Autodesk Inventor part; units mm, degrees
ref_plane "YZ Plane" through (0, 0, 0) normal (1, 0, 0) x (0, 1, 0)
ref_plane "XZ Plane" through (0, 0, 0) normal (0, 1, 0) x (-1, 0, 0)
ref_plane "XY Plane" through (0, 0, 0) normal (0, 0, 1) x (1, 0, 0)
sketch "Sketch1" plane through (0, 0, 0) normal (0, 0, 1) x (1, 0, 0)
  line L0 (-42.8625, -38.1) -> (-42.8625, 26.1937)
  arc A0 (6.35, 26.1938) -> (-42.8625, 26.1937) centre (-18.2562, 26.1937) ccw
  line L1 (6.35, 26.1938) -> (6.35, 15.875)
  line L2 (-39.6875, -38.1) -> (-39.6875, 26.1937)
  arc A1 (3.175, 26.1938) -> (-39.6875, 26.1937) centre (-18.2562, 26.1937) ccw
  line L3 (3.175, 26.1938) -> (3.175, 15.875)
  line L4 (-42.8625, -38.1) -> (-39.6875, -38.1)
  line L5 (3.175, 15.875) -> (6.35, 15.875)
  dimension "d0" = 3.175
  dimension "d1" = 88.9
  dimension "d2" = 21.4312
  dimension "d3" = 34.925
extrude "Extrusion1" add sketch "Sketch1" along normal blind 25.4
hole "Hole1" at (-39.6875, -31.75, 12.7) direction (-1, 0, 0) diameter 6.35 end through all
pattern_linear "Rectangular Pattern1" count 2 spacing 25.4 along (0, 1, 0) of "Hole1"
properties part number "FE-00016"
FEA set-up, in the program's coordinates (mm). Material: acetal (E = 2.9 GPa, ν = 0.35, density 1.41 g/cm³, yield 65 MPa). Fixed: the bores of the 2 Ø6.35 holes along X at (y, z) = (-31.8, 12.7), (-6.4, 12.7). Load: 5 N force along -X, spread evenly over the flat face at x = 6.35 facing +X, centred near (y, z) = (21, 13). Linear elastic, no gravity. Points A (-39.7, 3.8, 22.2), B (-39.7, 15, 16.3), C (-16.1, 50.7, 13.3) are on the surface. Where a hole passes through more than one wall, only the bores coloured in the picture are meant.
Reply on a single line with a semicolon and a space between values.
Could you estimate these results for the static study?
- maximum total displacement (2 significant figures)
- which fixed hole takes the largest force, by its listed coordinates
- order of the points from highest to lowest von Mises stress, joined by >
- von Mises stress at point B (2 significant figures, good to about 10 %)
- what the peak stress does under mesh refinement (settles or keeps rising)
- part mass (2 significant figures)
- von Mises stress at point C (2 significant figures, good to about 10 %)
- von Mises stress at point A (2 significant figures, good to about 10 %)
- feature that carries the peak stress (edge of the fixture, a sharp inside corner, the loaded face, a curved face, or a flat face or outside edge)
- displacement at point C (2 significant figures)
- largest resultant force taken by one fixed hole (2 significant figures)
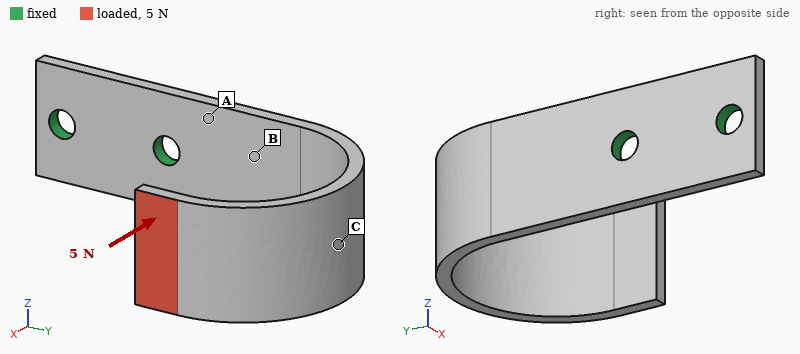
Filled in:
1.2 mm; (-6.4, 12.7); C > A > B; 0.63 MPa; keeps rising; 16 g; 2.7 MPa; 1.9 MPa; edge of the fixture; 0.26 mm; 5.6 N
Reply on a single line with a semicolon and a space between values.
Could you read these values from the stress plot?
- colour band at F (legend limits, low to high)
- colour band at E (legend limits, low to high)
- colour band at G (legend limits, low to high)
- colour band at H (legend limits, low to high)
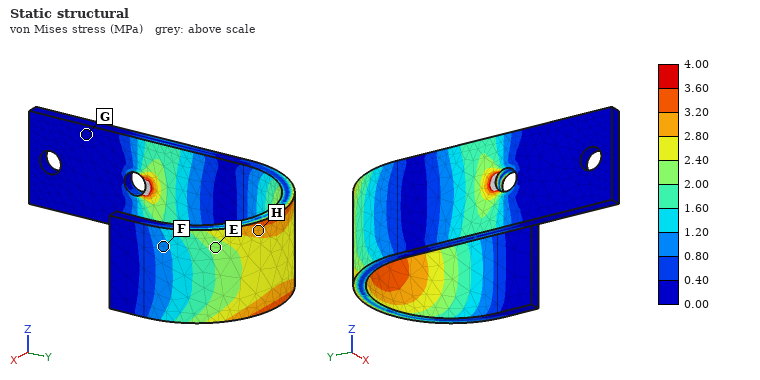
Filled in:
0.80 to 1.20 MPa; 2.00 to 2.40 MPa; 0.00 to 0.40 MPa; 2.80 to 3.20 MPa
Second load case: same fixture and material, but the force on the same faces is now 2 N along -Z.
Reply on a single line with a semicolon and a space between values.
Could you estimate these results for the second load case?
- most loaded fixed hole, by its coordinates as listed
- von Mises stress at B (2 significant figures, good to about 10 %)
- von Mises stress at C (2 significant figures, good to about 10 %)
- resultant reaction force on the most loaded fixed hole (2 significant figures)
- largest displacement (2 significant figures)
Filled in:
(-6.4, 12.7); 2.1 MPa; 1.1 MPa; 3.3 N; 1.1 mm
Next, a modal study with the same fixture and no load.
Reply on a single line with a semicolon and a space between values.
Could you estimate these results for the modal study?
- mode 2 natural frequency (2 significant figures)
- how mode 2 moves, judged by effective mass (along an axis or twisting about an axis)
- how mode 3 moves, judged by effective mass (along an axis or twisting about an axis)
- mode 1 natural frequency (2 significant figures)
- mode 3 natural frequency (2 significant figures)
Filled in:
120 Hz; along Z; along X; 85 Hz; 200 Hz
